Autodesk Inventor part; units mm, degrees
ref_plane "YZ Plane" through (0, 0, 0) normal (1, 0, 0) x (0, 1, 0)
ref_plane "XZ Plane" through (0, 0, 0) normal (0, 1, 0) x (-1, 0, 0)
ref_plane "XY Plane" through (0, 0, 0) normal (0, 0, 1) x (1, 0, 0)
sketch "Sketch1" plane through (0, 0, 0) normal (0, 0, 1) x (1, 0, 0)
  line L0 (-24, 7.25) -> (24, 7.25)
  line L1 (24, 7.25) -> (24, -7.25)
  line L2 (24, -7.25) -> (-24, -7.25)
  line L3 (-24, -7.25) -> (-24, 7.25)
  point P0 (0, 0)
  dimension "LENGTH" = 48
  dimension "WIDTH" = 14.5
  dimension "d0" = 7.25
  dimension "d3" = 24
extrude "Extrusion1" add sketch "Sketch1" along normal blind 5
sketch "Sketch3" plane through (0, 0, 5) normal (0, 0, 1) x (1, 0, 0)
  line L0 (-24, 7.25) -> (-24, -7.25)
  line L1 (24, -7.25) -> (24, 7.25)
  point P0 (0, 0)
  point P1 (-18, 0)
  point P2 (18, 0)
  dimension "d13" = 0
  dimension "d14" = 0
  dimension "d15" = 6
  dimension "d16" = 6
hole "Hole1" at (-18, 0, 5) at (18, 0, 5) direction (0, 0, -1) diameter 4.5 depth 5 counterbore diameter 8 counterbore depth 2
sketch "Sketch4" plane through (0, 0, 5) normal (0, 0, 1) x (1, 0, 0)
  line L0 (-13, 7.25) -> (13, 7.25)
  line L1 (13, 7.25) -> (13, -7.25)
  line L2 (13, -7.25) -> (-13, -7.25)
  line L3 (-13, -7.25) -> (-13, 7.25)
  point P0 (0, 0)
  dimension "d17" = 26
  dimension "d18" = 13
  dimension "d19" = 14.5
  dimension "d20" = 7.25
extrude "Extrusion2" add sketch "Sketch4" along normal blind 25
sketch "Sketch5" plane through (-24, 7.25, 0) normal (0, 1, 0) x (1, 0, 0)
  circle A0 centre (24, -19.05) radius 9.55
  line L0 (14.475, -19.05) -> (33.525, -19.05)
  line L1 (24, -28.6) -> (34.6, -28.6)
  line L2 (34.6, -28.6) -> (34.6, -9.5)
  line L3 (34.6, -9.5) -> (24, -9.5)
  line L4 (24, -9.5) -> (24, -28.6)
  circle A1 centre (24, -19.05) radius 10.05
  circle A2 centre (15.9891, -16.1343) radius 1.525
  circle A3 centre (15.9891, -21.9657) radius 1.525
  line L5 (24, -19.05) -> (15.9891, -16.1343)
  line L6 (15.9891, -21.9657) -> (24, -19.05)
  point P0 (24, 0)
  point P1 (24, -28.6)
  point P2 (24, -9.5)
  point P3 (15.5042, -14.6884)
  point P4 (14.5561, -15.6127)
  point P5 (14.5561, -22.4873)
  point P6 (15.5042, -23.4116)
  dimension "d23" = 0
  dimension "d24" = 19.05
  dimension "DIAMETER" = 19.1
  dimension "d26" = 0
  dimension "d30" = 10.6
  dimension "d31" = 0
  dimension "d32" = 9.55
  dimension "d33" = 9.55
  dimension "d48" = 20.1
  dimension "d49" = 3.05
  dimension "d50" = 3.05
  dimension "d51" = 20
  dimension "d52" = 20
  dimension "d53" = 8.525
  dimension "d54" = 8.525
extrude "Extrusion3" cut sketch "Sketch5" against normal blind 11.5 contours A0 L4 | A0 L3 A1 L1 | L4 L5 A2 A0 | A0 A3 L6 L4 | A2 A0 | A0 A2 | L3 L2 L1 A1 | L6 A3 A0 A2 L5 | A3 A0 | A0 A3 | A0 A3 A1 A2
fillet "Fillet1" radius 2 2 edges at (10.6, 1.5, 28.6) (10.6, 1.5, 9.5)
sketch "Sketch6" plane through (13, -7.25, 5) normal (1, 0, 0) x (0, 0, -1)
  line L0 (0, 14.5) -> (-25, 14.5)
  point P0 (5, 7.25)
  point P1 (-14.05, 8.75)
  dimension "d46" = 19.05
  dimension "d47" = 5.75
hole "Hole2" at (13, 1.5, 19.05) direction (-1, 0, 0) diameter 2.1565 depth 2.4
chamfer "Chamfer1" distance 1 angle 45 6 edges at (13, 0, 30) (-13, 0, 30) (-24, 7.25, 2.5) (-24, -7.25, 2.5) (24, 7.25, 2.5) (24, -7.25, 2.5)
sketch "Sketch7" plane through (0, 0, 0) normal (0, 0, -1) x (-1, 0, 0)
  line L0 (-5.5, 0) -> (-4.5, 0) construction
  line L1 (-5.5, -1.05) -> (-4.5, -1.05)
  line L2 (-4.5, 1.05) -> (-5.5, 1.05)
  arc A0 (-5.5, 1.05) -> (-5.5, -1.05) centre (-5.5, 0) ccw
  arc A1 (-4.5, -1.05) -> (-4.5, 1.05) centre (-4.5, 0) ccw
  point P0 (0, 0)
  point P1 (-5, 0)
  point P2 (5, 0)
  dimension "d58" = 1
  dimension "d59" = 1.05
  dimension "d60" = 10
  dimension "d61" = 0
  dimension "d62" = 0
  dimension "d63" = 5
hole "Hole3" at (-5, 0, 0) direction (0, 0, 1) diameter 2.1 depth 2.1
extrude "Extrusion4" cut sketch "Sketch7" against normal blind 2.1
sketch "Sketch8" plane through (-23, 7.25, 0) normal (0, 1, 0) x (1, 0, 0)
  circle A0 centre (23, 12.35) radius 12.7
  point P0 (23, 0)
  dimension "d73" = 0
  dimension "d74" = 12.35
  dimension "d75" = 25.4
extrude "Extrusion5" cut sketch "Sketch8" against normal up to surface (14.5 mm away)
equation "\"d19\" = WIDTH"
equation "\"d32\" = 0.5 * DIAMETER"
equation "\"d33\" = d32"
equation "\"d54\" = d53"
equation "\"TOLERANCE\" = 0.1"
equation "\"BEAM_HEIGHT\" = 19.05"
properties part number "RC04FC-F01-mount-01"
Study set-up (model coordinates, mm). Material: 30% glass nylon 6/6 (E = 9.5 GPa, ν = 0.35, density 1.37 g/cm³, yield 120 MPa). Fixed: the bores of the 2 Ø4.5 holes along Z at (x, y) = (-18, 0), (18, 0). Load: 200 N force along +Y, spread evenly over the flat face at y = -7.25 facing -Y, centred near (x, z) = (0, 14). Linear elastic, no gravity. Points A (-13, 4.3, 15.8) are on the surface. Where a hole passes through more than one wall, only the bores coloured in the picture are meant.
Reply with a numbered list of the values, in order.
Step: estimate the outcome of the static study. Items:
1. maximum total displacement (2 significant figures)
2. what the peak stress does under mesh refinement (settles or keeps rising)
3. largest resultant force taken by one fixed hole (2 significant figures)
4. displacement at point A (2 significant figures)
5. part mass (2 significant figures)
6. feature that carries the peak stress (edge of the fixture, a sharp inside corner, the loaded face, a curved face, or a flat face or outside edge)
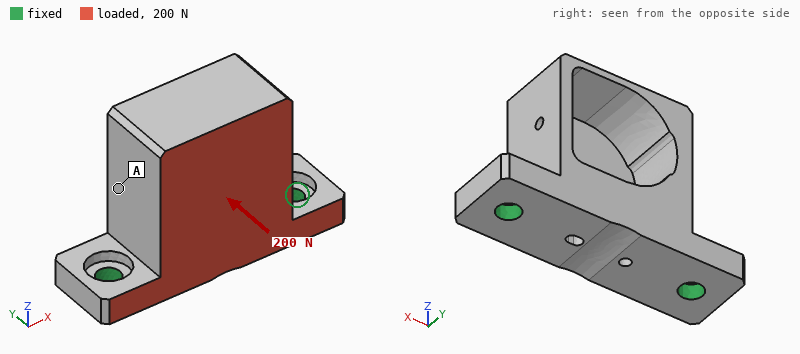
1. 0.19 mm
2. keeps rising
3. 100 N
4. 0.093 mm
5. 12 g
6. edge of the fixture
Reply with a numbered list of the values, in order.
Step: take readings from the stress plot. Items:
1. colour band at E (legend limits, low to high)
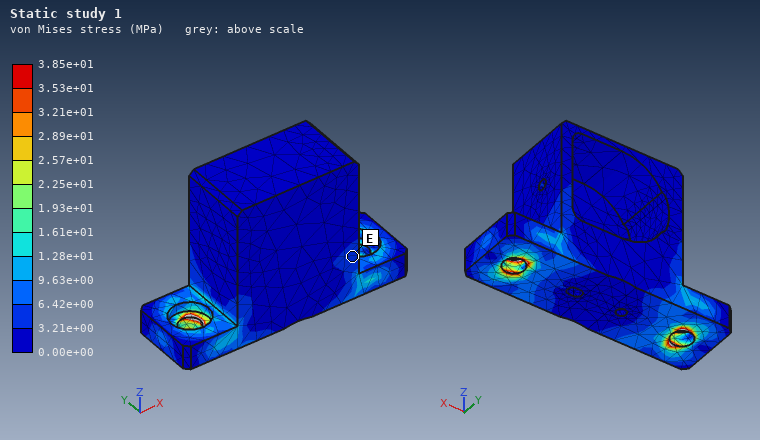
1. 3.21e+00 to 6.42e+00 MPa
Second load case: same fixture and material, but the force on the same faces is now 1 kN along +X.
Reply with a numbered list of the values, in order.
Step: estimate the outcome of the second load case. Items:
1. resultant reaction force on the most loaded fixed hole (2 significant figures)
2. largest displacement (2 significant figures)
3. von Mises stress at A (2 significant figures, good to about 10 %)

1. 670 N
2. 95 µm
3. 6.3 MPa
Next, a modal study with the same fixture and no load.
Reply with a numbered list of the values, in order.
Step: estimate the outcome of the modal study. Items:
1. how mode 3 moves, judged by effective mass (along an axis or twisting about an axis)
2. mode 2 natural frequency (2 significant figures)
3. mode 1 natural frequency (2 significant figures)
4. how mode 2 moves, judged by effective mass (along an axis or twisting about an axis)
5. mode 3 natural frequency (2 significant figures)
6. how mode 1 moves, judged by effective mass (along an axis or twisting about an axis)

1. along Z
2. 4900 Hz
3. 2000 Hz
4. along X
5. 7800 Hz
6. along Y
